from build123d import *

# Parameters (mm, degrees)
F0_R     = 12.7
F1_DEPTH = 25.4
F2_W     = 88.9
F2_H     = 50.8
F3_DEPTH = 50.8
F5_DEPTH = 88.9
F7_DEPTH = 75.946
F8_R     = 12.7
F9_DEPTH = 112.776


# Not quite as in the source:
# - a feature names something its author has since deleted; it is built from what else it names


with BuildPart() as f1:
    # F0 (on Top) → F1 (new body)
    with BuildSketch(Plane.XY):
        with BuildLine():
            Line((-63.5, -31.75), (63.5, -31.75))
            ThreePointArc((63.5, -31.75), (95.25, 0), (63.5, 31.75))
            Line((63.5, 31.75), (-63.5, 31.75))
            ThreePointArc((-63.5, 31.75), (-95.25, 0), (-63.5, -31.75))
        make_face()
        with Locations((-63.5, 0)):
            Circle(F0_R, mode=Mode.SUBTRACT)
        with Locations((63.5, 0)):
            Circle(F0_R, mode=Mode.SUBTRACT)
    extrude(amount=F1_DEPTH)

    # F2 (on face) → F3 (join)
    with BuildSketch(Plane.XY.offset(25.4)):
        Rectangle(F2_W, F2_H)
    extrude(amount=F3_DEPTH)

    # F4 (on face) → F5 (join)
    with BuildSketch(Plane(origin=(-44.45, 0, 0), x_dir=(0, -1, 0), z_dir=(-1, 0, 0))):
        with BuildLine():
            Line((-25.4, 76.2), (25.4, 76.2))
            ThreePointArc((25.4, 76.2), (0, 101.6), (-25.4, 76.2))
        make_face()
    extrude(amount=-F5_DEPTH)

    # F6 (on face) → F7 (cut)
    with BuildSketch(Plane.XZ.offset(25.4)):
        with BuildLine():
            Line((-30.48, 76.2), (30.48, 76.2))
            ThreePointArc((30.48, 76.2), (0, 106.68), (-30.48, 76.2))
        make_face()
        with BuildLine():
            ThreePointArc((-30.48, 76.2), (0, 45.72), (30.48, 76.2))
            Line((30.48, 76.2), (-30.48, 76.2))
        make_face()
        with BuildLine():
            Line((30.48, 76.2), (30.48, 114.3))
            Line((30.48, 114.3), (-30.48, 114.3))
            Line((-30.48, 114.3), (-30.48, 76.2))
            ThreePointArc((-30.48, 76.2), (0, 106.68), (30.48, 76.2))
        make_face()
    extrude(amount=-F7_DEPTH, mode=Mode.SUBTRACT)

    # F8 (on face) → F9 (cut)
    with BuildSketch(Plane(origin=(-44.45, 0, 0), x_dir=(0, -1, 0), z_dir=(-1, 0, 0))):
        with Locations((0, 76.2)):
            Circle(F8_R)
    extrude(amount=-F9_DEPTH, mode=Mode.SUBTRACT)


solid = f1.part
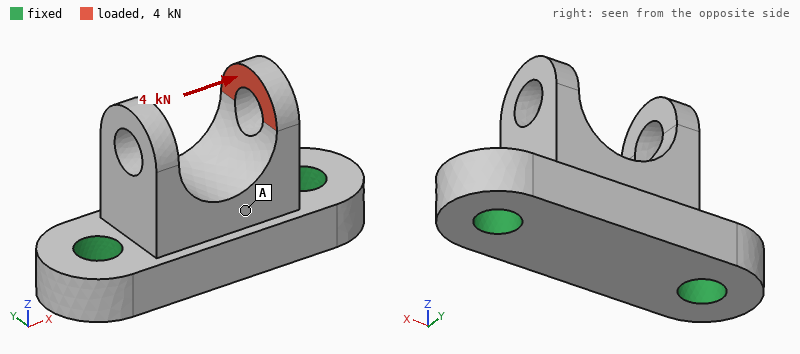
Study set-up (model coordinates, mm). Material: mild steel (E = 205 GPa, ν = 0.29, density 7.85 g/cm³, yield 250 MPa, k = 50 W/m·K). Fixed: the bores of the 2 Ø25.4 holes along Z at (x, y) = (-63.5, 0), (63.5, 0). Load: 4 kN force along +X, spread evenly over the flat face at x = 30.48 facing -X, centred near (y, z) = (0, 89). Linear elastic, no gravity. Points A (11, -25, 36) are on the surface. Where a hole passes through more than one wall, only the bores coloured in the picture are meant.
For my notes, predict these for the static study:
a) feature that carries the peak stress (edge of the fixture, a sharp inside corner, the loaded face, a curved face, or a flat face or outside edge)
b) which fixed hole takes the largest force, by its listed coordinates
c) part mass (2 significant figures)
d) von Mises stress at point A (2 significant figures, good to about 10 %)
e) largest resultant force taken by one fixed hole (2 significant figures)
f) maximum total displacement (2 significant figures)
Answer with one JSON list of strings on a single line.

["a curved face", "(-63.5, 0)", "3.4 kg", "7.7 MPa", "4.4 kN", "64 µm"]
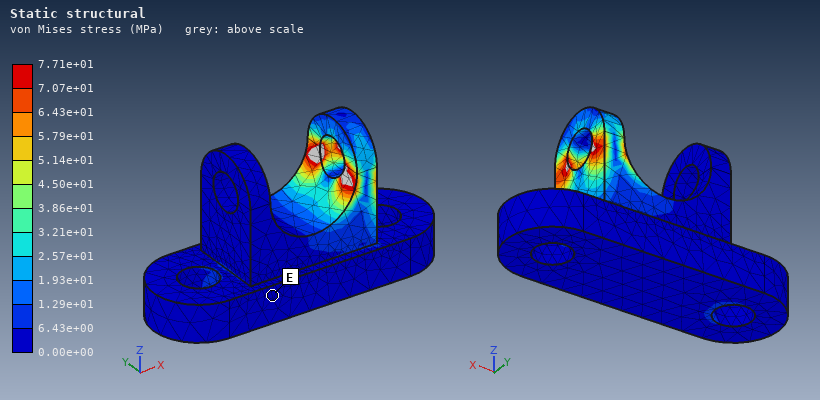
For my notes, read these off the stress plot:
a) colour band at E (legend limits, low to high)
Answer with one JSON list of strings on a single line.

["0.00e+00 to 6.43e+00 MPa"]
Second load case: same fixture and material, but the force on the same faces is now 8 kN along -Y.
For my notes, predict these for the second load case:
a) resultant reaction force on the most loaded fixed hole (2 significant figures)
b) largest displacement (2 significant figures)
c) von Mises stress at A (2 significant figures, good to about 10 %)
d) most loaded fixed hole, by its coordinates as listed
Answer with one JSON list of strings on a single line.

["6.0 kN", "73 µm", "18 MPa", "(63.5, 0)"]
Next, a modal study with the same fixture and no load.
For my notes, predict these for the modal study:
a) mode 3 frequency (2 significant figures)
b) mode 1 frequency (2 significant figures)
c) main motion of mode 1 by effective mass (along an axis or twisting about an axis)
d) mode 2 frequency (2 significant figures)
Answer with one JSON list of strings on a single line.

["5000 Hz", "3900 Hz", "along Y", "5000 Hz"]
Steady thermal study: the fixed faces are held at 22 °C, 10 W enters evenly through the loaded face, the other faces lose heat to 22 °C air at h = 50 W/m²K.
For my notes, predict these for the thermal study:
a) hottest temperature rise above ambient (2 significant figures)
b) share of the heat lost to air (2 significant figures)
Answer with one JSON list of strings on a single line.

["19 K", "43 %"]
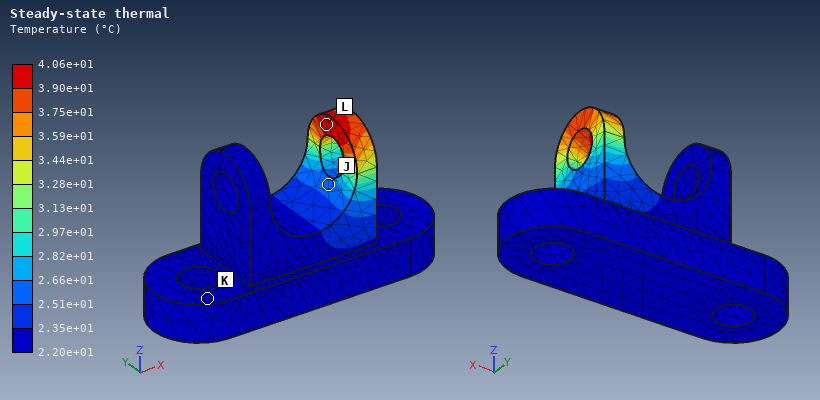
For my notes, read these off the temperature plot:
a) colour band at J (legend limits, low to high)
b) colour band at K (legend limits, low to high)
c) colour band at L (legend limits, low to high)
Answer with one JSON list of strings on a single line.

["2.51e+01 to 2.66e+01 °C", "2.20e+01 to 2.35e+01 °C", "3.90e+01 to 4.06e+01 °C"]
